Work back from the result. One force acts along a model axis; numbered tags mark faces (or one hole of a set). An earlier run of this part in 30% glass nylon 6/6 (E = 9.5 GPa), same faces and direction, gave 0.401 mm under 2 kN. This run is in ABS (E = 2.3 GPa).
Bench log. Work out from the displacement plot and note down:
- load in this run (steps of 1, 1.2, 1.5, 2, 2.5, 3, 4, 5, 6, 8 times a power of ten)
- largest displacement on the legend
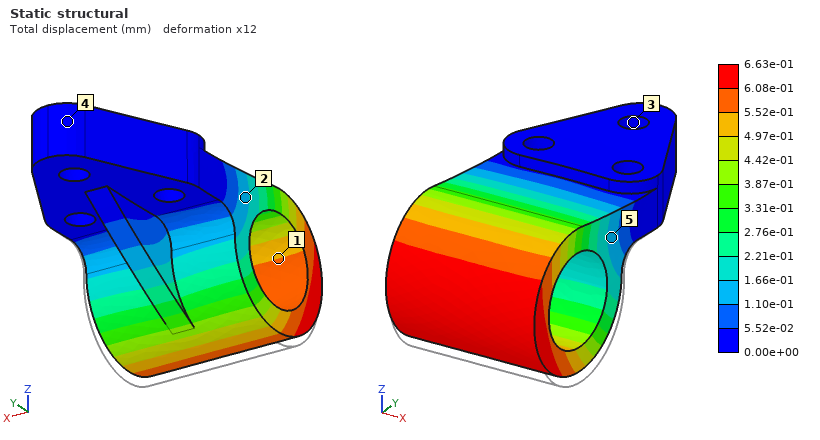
800 N
6.63e-01 mm
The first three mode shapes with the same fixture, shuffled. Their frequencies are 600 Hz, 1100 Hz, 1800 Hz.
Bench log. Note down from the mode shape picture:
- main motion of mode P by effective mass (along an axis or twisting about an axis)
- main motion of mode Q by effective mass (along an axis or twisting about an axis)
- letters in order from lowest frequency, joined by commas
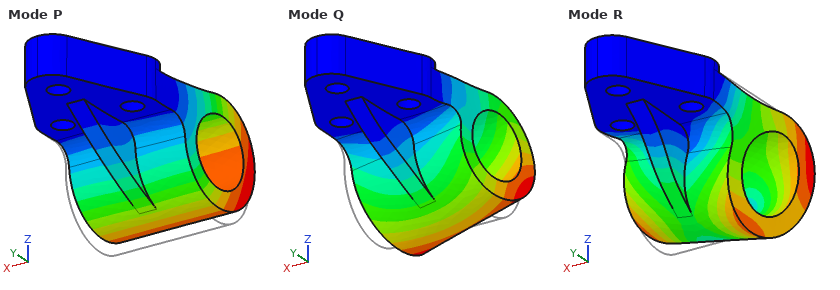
along Z
along X
P, Q, R
